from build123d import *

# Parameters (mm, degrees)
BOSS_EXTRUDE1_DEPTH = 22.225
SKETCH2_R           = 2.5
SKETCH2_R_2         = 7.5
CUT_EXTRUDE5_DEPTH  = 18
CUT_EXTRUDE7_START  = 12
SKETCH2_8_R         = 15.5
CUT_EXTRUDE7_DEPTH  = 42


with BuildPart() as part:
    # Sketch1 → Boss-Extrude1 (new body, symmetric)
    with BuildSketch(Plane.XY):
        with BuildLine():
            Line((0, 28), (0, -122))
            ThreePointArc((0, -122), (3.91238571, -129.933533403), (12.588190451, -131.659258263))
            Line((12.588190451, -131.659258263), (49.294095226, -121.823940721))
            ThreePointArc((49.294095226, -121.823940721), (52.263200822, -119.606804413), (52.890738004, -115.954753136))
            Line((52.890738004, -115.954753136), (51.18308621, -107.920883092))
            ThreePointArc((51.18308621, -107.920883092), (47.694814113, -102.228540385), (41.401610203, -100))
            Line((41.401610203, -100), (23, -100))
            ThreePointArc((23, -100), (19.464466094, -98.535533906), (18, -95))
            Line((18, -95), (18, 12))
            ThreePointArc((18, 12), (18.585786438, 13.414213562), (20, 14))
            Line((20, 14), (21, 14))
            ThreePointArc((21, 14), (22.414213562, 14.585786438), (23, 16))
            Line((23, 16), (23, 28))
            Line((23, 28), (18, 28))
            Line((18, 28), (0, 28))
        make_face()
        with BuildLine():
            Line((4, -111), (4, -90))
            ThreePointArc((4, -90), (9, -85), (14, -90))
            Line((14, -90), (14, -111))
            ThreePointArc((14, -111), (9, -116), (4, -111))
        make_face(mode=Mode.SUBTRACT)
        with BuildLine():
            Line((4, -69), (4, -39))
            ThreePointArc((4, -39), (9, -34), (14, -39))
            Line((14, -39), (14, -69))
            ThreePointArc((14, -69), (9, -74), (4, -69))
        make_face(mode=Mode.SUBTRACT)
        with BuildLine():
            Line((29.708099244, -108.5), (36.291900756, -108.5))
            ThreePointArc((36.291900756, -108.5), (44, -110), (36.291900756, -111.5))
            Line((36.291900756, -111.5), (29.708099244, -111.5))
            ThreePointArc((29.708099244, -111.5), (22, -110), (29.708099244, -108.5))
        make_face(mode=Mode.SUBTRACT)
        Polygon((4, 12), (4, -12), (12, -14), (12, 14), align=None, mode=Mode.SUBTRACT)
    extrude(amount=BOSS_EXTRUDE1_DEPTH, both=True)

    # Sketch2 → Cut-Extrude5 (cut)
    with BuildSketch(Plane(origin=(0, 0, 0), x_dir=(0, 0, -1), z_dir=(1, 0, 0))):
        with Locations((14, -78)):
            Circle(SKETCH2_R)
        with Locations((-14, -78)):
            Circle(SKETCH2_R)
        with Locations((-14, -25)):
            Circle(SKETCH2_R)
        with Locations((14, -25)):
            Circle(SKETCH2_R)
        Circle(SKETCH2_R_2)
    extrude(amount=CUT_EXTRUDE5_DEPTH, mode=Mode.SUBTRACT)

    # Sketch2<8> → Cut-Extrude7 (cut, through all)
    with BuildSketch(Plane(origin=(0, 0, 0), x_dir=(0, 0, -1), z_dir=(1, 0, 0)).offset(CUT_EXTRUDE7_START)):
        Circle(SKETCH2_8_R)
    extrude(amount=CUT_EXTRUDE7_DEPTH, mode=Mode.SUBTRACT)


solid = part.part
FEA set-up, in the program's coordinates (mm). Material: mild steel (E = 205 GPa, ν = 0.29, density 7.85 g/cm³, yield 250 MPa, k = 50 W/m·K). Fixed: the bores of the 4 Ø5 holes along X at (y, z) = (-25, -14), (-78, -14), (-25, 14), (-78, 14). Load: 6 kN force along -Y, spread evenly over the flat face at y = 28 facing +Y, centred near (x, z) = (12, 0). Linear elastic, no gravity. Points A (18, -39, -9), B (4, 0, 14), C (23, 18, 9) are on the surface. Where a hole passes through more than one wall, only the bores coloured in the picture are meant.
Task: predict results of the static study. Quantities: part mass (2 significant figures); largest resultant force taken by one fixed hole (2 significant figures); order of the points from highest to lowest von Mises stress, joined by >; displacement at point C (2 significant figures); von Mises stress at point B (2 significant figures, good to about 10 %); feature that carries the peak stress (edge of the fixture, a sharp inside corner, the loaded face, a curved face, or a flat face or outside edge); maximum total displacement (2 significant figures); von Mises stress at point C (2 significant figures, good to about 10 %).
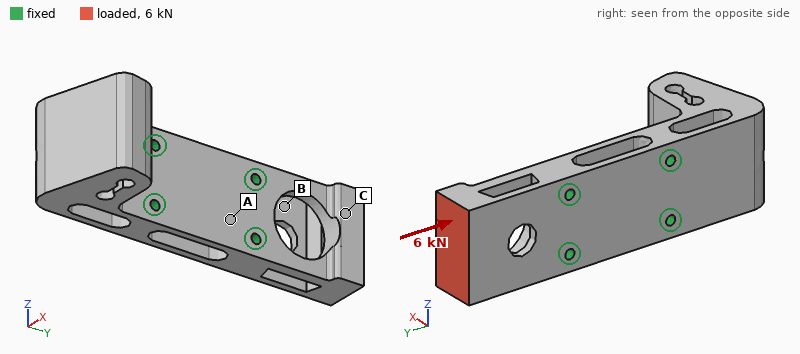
920 g
2.9 kN
B > C > A
19 µm
22 MPa
a curved face
24 µm
10 MPa
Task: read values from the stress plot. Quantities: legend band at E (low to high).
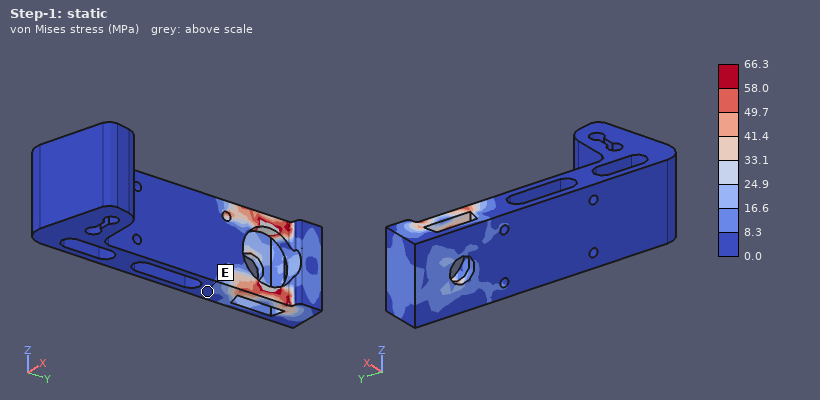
0.0 to 8.3 MPa
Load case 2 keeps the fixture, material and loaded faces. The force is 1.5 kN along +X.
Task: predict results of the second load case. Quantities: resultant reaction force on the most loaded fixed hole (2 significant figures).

790 N
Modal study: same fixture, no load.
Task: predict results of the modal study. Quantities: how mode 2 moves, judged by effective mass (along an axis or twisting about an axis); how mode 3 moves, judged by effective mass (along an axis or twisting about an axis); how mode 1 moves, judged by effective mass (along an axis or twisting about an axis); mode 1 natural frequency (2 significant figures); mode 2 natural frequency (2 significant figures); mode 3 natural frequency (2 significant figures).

along X
along Z
along X
1800 Hz
2400 Hz
2700 Hz
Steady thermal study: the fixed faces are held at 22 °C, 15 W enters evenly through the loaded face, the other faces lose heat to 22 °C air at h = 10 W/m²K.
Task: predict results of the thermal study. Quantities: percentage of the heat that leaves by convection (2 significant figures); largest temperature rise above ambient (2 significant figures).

13 %
42 K
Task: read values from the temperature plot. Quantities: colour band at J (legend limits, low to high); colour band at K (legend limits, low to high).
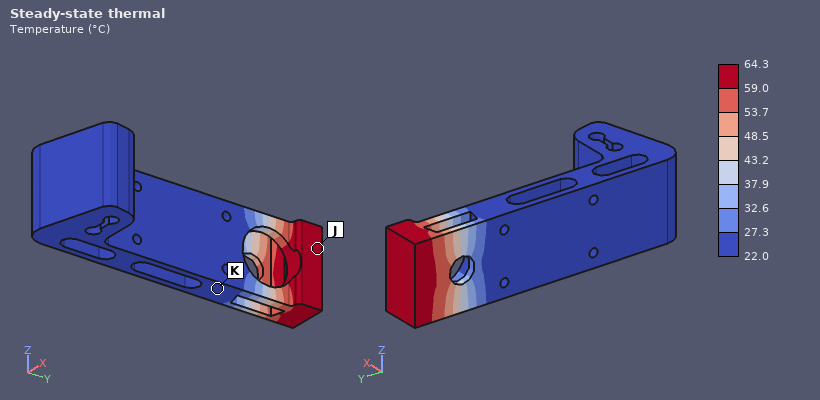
59.0 to 64.3 °C
22.0 to 27.3 °C
